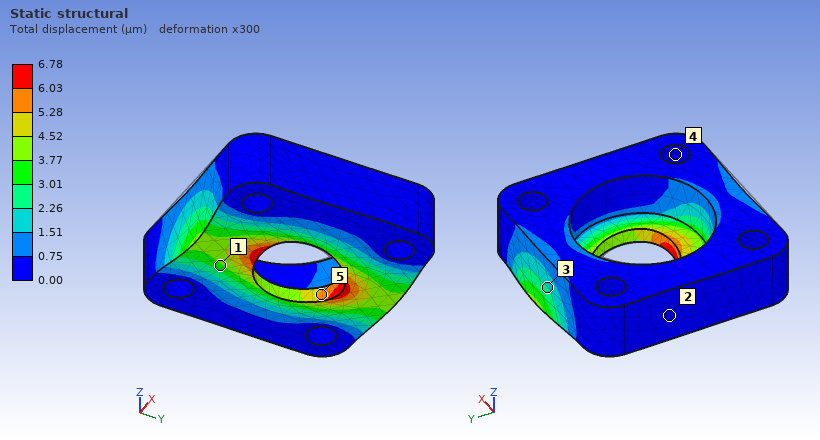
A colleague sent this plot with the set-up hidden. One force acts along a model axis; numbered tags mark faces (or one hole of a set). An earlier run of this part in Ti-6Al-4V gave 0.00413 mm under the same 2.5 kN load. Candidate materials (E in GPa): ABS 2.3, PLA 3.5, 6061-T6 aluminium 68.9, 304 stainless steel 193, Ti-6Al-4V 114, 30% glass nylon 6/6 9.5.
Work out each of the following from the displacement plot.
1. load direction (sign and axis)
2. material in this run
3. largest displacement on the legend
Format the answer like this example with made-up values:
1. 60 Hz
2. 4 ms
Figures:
1. +Y
2. 6061-T6 aluminium
3. 6.78 µm
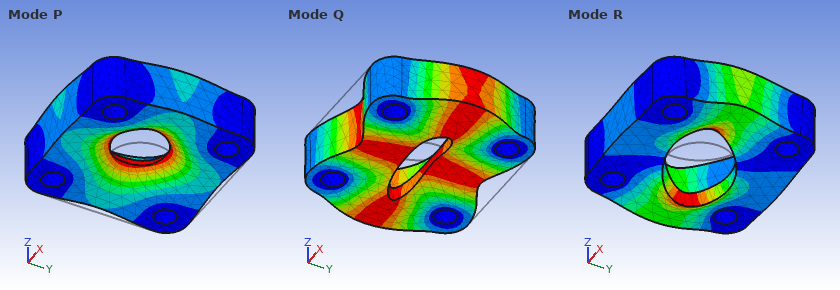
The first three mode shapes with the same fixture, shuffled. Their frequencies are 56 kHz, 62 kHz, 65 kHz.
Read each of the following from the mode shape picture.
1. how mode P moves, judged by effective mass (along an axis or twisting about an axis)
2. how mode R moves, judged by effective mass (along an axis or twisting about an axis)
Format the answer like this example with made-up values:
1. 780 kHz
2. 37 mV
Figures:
1. along Z
2. twisting about Y
